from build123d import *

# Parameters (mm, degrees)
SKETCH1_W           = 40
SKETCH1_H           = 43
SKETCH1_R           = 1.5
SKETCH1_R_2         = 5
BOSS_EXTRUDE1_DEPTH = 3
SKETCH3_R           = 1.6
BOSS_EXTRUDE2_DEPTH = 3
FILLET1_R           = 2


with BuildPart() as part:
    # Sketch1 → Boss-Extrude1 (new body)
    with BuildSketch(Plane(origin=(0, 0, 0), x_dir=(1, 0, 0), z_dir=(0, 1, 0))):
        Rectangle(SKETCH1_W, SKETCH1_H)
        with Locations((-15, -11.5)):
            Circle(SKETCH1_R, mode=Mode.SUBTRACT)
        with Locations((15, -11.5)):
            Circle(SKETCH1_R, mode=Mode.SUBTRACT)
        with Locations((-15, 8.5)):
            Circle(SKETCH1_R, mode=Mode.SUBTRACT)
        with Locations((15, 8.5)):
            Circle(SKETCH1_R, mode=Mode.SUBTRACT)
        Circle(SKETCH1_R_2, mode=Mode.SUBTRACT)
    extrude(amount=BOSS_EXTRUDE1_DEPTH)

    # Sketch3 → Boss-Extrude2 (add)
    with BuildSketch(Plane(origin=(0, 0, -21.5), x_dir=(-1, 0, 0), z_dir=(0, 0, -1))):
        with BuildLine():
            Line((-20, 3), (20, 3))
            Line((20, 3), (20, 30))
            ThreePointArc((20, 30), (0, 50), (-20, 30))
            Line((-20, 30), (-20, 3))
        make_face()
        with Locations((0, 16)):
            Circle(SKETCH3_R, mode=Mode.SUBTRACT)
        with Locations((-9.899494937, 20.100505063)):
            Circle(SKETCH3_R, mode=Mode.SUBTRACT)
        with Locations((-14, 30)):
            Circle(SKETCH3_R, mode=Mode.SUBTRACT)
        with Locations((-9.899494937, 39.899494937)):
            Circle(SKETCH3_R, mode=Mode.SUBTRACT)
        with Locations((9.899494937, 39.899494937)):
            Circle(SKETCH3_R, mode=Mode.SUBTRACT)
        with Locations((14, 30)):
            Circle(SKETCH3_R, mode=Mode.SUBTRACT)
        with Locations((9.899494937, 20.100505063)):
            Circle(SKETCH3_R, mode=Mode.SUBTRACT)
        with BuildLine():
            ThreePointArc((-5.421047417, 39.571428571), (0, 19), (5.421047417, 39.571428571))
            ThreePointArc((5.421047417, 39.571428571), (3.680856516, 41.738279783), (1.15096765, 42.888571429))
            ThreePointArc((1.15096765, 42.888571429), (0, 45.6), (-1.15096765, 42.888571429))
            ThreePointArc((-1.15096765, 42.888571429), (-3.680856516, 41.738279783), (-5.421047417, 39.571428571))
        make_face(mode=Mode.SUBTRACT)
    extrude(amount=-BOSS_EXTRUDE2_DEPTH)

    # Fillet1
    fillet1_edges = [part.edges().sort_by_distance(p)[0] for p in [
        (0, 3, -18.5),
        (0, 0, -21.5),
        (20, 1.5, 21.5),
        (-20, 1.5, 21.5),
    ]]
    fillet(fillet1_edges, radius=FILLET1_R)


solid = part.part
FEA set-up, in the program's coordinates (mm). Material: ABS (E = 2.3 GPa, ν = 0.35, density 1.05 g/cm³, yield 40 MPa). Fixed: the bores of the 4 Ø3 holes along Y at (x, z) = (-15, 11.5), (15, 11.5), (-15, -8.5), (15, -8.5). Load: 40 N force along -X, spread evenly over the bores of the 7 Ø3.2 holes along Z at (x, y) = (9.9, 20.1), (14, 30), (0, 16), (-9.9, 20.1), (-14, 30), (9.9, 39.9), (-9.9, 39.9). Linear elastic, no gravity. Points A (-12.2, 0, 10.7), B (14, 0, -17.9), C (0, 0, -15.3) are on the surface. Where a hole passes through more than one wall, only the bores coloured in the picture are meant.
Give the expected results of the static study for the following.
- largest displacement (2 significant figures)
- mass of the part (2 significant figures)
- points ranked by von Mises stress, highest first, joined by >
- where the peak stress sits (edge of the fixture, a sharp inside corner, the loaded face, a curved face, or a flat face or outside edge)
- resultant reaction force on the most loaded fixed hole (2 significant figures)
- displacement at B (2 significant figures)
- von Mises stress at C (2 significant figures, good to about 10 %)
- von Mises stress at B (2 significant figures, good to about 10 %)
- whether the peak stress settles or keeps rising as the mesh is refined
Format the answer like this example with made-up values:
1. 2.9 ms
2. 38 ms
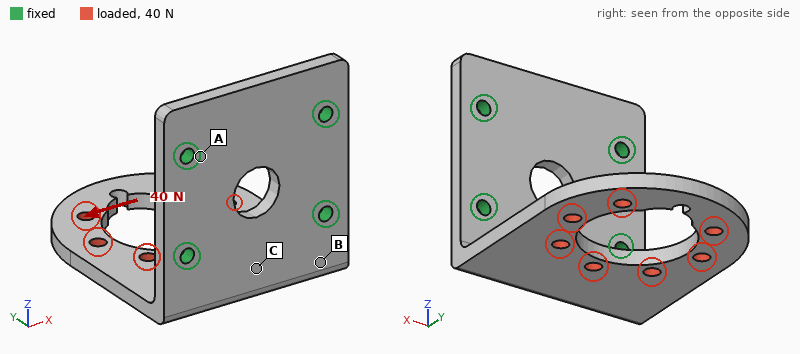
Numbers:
1. 0.45 mm
2. 9.0 g
3. B > C > A
4. edge of the fixture
5. 43 N
6. 0.087 mm
7. 2.5 MPa
8. 3.7 MPa
9. keeps rising
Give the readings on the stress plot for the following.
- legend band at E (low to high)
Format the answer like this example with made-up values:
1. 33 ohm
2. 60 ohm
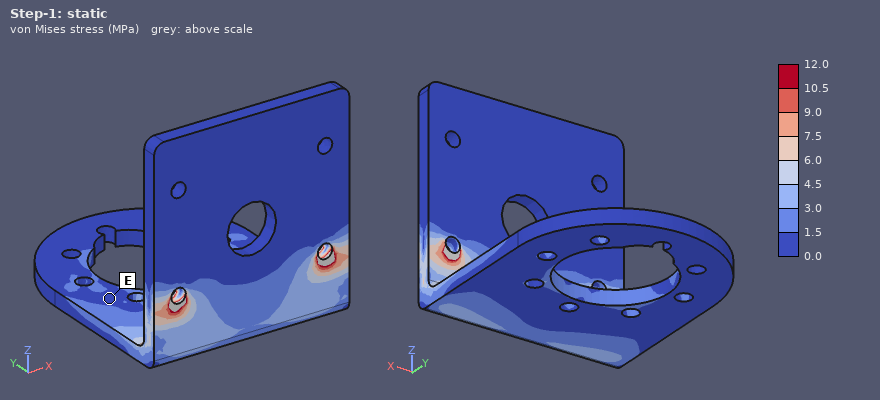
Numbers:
1. 0.0 to 1.5 MPa
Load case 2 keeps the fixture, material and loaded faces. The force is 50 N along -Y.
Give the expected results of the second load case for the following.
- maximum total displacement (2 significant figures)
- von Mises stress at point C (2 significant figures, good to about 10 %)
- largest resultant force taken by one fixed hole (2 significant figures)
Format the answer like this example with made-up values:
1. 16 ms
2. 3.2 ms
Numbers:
1. 0.85 mm
2. 2.6 MPa
3. 29 N
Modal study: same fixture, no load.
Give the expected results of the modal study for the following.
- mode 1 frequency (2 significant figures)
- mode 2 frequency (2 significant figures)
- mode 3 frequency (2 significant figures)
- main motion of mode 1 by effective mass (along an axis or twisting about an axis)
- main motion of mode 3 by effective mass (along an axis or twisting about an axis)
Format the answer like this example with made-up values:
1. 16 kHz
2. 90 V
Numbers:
1. 300 Hz
2. 800 Hz
3. 1100 Hz
4. along Z
5. along X
